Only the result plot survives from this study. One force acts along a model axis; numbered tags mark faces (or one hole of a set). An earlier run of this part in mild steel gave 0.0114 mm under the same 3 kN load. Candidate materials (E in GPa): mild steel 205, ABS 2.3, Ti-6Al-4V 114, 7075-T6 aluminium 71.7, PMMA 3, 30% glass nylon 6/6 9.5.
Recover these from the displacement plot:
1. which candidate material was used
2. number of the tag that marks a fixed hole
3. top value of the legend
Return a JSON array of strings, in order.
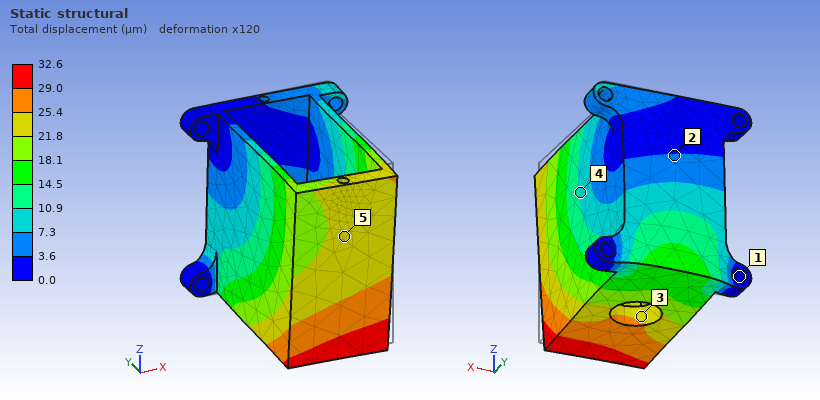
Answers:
["7075-T6 aluminium", "1", "32.6 µm"]
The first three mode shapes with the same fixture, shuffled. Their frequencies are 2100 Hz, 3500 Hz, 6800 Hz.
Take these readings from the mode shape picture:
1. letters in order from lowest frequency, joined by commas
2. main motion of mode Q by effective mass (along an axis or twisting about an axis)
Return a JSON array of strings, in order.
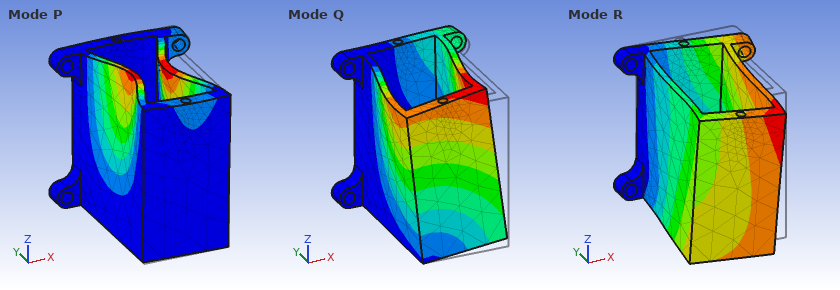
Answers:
["Q, R, P", "along X"]
